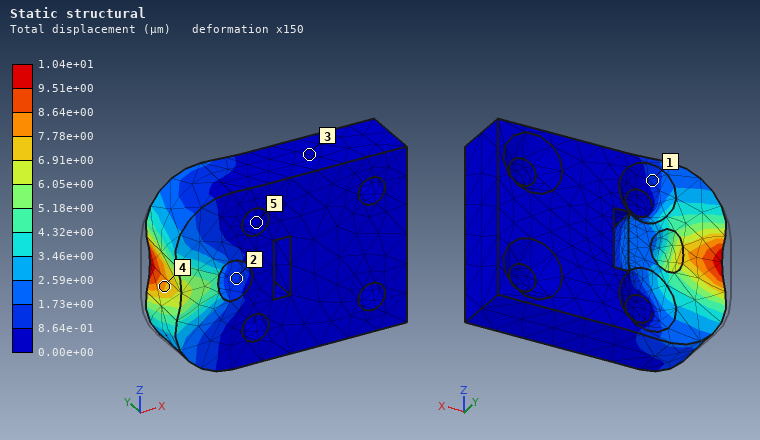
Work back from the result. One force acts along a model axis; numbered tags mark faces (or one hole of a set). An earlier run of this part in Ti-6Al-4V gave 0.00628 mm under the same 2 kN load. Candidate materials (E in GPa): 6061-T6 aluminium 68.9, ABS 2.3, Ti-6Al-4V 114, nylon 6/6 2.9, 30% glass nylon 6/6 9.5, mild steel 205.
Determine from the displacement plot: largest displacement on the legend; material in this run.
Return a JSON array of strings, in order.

["1.04e+01 µm", "6061-T6 aluminium"]
